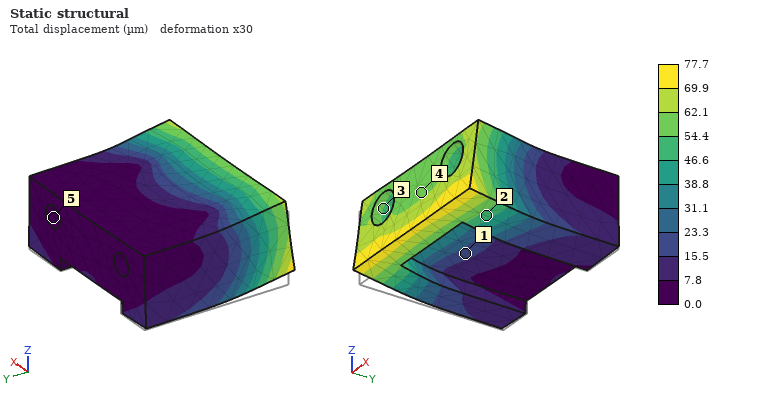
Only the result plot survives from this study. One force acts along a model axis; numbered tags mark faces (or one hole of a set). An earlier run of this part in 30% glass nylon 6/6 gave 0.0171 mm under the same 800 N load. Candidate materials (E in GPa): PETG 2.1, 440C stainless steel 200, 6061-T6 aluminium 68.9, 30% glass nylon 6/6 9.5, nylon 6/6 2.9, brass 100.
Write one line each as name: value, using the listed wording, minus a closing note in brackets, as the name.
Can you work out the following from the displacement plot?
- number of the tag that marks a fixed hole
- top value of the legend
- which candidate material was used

number of the tag that marks a fixed hole: 5
top value of the legend: 77.7 µm
which candidate material was used: PETG
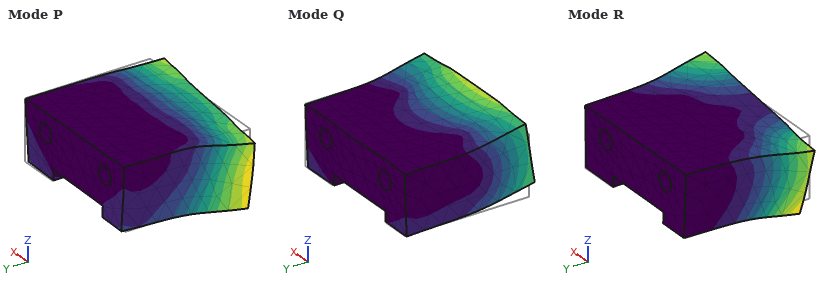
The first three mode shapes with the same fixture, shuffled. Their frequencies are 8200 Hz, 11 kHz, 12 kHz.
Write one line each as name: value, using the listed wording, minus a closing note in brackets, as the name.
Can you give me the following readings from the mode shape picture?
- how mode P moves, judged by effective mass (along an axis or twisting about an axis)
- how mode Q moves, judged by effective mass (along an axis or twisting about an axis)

how mode P moves, judged by effective mass: along X
how mode Q moves, judged by effective mass: along Z
